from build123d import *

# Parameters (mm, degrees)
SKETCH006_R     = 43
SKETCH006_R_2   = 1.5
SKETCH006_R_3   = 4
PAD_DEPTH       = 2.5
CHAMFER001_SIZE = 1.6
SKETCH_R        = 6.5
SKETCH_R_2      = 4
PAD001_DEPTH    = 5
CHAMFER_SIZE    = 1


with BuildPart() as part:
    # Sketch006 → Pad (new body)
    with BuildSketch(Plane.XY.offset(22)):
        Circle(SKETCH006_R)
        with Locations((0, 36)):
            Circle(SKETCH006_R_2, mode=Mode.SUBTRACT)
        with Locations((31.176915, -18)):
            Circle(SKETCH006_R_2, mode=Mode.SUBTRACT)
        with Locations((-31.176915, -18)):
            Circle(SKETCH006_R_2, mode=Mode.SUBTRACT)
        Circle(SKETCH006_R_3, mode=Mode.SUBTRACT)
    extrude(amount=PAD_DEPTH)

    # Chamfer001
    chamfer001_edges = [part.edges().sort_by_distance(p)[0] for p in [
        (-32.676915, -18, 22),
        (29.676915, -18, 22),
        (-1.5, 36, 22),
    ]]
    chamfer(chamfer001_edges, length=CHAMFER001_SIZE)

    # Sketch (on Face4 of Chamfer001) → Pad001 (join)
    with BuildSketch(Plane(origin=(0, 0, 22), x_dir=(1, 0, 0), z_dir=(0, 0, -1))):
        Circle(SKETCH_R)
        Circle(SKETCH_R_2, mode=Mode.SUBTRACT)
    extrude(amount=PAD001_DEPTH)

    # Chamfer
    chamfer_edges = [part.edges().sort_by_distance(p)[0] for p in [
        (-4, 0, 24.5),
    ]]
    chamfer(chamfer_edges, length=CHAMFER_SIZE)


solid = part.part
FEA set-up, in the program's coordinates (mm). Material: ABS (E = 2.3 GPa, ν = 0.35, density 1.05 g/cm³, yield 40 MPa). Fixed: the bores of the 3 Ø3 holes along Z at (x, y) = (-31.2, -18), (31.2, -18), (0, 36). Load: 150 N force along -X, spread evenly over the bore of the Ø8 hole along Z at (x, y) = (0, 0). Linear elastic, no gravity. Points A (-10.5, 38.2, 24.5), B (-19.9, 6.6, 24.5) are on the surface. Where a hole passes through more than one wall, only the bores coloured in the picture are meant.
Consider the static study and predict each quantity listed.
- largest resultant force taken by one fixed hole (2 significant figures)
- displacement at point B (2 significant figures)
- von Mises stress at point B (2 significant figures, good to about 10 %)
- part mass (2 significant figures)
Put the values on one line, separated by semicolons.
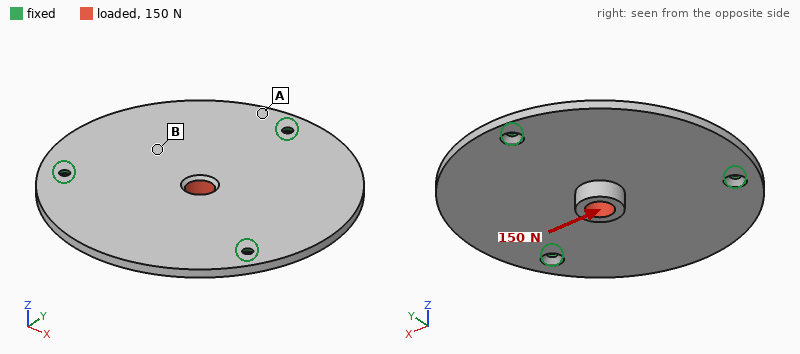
62 N; 0.16 mm; 1.8 MPa; 15 g
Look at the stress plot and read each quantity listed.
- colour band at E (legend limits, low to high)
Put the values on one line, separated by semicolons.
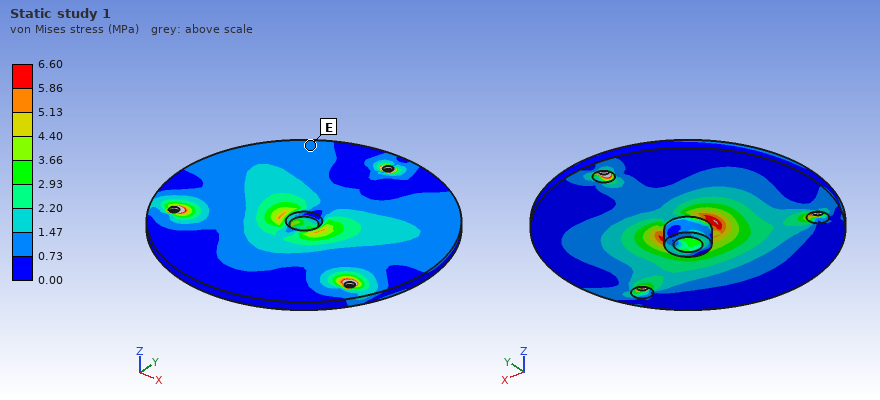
0.73 to 1.47 MPa
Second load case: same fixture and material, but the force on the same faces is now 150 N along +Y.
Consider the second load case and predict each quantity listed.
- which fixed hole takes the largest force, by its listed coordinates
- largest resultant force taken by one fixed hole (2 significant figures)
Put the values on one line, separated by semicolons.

(0, 36); 70 N
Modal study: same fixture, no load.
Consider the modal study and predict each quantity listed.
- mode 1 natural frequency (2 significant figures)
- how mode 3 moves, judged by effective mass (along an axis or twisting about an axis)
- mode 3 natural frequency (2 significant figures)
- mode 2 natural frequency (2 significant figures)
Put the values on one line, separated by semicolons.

530 Hz; along Z; 630 Hz; 530 Hz
